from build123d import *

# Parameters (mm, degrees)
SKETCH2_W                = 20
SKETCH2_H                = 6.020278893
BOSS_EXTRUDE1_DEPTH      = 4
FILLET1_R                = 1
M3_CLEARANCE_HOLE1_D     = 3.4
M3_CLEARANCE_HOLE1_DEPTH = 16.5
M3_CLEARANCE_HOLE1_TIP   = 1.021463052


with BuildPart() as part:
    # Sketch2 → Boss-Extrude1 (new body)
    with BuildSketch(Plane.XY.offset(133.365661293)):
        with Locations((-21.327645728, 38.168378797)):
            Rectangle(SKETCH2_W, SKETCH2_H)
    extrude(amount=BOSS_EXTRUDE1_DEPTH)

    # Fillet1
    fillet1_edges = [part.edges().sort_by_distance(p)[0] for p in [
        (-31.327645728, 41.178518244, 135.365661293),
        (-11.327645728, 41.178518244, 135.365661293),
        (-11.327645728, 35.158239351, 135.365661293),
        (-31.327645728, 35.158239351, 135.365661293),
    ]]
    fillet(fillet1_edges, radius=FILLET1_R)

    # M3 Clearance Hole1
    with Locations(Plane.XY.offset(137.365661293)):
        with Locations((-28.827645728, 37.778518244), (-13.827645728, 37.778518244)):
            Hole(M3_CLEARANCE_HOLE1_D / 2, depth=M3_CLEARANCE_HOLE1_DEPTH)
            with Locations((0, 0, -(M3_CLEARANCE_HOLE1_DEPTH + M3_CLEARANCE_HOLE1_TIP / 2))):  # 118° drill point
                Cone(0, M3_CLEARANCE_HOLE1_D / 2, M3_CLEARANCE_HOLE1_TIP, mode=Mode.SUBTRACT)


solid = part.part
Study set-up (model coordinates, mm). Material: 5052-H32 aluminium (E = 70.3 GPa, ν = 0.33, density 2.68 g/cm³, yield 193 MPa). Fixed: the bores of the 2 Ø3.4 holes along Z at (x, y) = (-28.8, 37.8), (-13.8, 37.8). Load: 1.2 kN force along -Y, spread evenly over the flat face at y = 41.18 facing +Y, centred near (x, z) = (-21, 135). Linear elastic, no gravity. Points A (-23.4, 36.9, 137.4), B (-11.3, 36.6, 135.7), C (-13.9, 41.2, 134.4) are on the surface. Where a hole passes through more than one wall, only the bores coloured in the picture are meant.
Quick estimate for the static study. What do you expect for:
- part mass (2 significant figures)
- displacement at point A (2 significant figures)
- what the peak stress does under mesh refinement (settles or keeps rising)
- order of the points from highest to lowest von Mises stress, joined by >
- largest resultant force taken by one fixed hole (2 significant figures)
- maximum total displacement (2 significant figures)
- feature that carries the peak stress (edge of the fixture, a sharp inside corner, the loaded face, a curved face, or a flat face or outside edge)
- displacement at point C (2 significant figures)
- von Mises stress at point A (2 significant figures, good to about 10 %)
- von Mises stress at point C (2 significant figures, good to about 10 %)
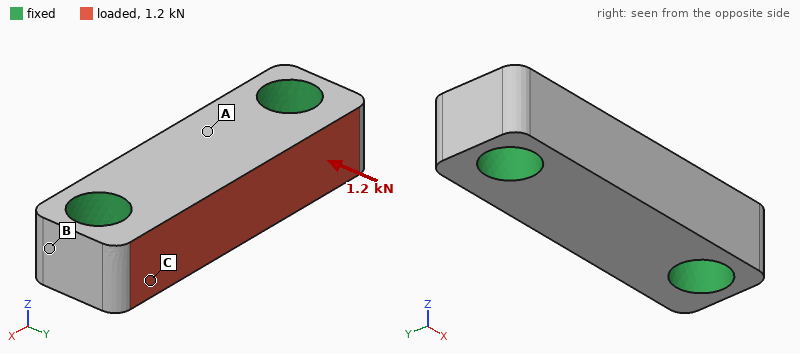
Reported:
1.1 g
3.3 µm
keeps rising
C > A > B
610 N
4.3 µm
edge of the fixture
0.77 µm
15 MPa
27 MPa
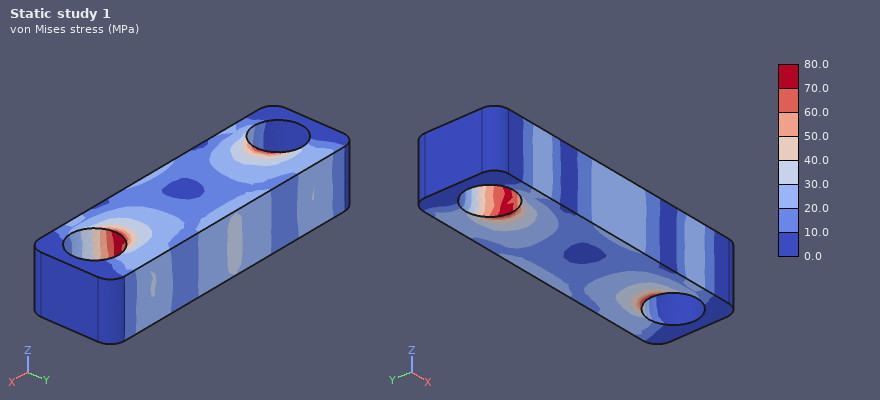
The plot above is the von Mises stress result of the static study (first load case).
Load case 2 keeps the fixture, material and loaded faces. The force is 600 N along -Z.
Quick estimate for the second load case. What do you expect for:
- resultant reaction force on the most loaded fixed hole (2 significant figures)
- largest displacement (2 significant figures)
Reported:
300 N
6.9 µm
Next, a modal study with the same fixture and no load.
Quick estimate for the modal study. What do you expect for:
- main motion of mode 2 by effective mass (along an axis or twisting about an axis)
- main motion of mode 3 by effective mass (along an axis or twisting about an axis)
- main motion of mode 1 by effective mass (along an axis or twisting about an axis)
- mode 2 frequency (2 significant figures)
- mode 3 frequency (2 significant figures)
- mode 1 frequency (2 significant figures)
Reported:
along Y
twisting about X
along Z
92 kHz
110 kHz
86 kHz
